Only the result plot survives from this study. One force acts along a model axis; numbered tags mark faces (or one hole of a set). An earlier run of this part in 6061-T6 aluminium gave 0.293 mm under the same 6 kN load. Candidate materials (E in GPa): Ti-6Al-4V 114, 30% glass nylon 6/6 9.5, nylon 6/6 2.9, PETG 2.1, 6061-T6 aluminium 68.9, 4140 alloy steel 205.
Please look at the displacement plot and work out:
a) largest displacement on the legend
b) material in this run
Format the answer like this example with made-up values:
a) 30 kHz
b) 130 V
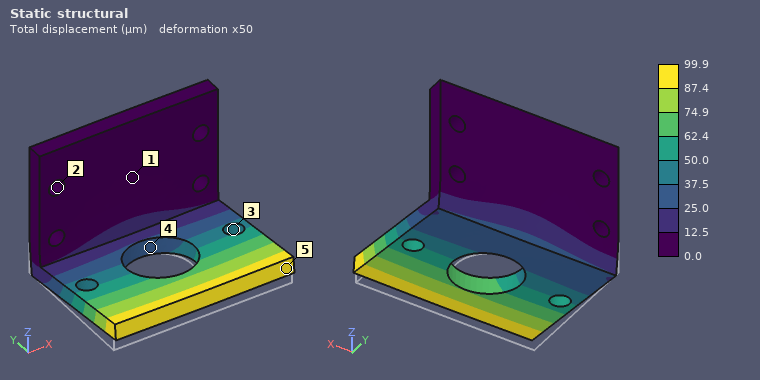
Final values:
a) 99.9 µm
b) 4140 alloy steel
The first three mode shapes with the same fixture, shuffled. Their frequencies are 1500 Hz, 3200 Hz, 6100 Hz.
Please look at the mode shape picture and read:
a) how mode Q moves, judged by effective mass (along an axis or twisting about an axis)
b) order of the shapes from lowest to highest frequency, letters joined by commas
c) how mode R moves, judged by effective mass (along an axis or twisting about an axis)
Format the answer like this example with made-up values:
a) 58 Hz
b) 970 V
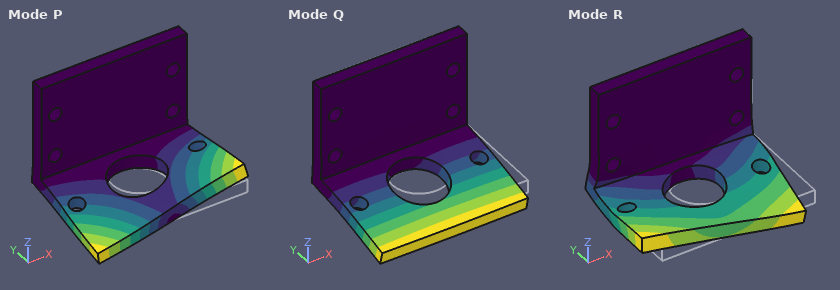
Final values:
a) along Z
b) Q, P, R
c) along X
